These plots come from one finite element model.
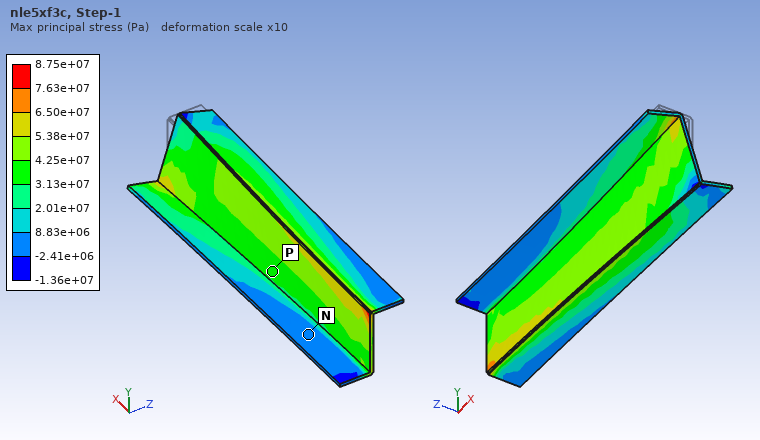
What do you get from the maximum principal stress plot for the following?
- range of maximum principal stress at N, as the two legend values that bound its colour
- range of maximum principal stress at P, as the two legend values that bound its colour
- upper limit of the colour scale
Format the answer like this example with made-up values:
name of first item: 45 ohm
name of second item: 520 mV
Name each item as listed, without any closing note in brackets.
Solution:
range of maximum principal stress at N, as the two legend values that bound its colour: -2.41e+06 to 8.83e+06 Pa
range of maximum principal stress at P, as the two legend values that bound its colour: 3.13e+07 to 4.25e+07 Pa
upper limit of the colour scale: 8.75e+07 Pa
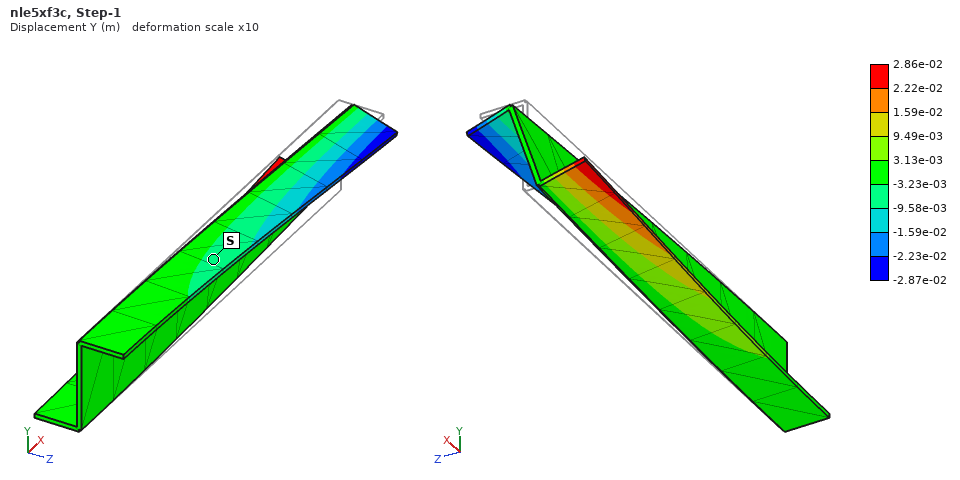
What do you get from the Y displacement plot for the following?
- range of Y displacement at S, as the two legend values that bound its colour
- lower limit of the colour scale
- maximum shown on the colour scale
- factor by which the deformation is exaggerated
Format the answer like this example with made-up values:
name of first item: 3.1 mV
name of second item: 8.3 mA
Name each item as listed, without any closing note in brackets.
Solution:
range of Y displacement at S, as the two legend values that bound its colour: -9.58e-03 to -3.23e-03 m
lower limit of the colour scale: -2.87e-02 m
maximum shown on the colour scale: 2.86e-02 m
factor by which the deformation is exaggerated: 10
